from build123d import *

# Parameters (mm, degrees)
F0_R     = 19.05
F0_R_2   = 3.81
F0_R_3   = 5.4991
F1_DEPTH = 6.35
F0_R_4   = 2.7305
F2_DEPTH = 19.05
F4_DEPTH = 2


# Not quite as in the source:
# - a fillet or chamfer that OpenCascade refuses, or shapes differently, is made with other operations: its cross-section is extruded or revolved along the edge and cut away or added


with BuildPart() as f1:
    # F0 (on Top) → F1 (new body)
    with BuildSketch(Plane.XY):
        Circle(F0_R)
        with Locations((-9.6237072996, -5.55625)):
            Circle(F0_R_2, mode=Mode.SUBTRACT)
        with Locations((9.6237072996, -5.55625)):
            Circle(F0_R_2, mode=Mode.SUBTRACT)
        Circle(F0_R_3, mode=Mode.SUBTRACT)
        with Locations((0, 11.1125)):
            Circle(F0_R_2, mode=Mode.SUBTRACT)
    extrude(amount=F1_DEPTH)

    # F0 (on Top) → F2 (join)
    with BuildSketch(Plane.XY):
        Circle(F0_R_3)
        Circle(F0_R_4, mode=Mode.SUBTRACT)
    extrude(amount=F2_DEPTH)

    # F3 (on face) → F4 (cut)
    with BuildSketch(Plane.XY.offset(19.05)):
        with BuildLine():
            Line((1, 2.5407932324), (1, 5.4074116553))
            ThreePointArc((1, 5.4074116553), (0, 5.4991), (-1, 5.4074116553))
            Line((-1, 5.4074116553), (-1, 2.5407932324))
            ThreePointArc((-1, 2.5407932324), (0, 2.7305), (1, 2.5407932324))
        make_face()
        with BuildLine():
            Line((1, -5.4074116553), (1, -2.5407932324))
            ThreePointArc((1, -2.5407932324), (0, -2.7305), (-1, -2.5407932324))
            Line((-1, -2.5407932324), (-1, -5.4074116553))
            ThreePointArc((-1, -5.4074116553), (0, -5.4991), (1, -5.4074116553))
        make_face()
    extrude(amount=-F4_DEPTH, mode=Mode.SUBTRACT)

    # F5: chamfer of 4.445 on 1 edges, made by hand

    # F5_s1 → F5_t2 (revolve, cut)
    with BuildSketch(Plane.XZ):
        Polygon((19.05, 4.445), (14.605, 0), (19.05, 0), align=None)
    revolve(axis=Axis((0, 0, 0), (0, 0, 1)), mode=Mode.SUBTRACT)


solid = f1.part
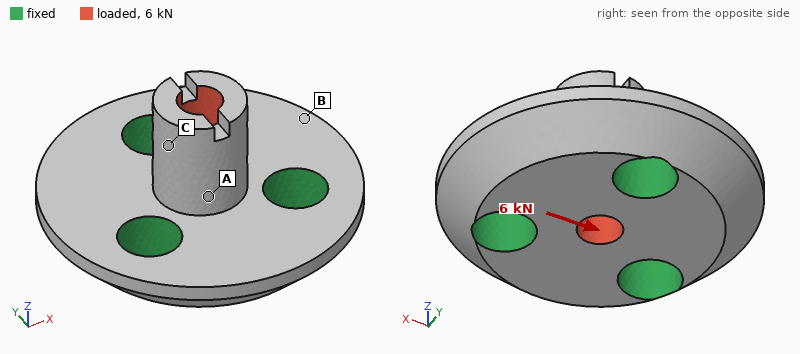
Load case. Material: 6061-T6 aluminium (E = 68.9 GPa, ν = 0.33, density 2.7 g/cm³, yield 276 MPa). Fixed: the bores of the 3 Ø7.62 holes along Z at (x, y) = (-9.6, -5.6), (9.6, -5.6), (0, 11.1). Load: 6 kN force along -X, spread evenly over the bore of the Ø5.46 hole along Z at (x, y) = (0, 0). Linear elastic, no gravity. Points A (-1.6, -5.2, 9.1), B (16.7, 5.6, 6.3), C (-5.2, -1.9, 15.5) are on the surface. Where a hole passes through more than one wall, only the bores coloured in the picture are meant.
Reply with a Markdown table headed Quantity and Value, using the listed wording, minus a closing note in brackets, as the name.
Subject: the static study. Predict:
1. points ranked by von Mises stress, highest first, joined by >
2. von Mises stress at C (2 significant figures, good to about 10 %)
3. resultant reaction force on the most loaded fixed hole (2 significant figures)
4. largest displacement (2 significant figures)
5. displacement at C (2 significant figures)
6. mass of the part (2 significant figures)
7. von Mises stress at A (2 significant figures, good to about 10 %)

| Quantity | Value |
|---|---|
| points ranked by von Mises stress, highest first, joined by > | A > C > B |
| von Mises stress at C | 30 MPa |
| resultant reaction force on the most loaded fixed hole | 3.1 kN |
| largest displacement | 70 µm |
| displacement at C | 54 µm |
| mass of the part | 16 g |
| von Mises stress at A | 95 MPa |
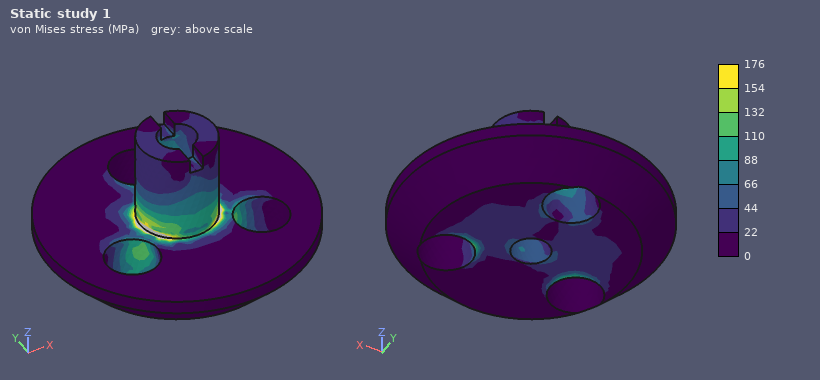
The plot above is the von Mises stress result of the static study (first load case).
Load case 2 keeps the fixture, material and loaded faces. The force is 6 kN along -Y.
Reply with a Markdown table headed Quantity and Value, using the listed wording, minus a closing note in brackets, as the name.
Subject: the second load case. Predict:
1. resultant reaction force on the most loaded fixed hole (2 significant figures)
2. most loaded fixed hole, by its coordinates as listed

| Quantity | Value |
|---|---|
| resultant reaction force on the most loaded fixed hole | 3.4 kN |
| most loaded fixed hole, by its coordinates as listed | (0, 11.1) |
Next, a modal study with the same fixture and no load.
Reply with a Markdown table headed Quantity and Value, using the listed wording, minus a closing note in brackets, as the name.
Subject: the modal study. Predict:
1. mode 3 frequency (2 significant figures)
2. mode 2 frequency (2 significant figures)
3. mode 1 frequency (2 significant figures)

| Quantity | Value |
|---|---|
| mode 3 frequency | 44 kHz |
| mode 2 frequency | 29 kHz |
| mode 1 frequency | 29 kHz |
